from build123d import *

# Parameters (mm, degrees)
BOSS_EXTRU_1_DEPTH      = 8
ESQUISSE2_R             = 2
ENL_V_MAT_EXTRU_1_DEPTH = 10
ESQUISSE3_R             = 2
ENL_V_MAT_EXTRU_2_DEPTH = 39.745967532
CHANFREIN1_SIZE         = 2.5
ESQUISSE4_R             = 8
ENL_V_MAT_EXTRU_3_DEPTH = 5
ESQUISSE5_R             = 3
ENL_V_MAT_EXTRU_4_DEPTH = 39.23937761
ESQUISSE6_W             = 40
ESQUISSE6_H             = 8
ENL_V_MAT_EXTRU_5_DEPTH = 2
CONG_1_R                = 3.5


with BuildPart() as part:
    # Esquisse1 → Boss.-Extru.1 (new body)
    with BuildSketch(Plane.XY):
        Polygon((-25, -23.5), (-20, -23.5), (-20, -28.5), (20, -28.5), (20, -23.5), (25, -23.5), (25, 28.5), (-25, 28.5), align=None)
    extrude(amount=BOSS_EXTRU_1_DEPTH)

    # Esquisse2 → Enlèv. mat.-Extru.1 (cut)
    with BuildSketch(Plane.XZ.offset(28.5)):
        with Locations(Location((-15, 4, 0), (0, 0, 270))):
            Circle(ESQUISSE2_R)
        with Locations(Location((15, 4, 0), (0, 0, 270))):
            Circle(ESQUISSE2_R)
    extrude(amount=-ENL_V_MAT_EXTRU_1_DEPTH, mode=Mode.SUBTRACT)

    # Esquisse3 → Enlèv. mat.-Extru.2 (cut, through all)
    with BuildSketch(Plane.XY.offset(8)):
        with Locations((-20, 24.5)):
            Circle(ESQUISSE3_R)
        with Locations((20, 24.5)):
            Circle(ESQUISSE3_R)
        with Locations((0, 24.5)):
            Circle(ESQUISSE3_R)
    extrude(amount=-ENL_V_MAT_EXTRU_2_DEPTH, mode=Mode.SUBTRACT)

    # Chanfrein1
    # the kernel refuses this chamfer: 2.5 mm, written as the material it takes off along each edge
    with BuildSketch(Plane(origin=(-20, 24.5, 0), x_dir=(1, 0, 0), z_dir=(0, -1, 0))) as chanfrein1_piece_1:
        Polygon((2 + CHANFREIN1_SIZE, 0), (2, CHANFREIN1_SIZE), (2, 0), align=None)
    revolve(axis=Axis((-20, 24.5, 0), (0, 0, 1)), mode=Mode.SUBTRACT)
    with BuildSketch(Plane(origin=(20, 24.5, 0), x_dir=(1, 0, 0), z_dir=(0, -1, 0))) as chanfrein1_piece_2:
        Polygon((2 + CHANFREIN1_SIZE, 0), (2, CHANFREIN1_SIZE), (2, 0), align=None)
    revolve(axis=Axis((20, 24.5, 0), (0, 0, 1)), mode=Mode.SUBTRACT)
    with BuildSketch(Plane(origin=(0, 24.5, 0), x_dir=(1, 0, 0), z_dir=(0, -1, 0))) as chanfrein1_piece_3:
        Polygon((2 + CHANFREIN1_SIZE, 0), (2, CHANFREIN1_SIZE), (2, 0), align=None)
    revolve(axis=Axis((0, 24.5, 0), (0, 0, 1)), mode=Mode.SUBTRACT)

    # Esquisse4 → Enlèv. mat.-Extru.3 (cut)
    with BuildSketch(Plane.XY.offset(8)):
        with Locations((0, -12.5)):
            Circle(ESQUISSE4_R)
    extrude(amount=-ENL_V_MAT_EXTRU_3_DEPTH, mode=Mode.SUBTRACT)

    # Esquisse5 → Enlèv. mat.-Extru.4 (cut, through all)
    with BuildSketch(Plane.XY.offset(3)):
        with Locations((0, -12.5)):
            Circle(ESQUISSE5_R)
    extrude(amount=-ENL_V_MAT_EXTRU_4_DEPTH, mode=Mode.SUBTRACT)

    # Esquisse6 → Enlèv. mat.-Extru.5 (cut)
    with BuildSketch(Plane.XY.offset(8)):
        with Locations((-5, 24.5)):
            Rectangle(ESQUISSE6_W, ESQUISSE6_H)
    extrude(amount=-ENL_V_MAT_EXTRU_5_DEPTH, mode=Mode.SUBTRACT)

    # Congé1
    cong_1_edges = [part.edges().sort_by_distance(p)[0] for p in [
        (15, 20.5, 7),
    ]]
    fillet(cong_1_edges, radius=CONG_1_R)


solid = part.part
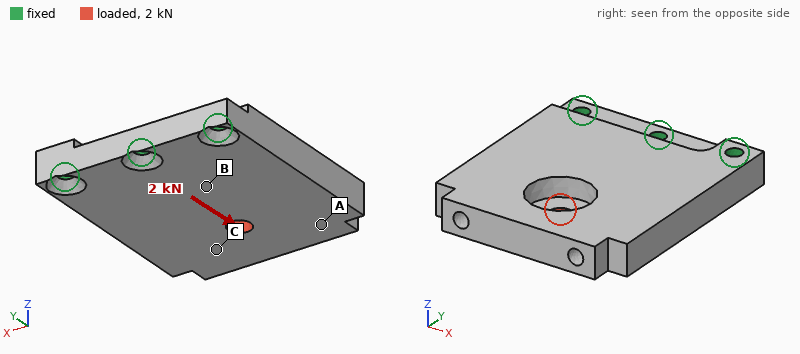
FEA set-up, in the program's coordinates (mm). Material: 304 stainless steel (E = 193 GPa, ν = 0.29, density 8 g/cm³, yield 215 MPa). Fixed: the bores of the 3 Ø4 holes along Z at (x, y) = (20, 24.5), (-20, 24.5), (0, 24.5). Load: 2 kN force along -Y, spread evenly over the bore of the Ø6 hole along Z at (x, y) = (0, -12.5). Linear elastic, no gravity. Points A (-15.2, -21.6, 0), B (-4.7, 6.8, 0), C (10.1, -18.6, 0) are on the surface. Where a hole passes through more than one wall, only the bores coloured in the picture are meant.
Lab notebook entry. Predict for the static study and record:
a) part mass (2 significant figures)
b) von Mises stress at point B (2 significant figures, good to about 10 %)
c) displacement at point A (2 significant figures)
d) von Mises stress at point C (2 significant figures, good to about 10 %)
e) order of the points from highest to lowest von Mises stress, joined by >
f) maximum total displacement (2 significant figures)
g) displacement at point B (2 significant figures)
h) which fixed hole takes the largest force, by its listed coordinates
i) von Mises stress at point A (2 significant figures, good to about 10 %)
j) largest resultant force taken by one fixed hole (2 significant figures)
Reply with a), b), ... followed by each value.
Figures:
a) 160 g
b) 15 MPa
c) 20 µm
d) 11 MPa
e) B > C > A
f) 25 µm
g) 5.7 µm
h) (0, 24.5)
i) 5.5 MPa
j) 770 N
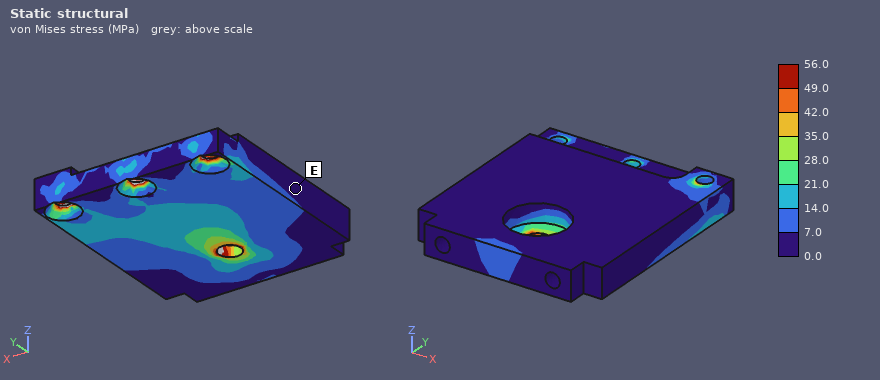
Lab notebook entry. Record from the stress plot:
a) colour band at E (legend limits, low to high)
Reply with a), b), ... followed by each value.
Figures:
a) 0.0 to 7.0 MPa
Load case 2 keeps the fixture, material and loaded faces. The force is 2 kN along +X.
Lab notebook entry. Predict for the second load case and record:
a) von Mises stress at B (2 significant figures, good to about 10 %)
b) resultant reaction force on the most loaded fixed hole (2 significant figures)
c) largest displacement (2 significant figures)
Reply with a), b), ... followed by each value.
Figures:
a) 18 MPa
b) 2.0 kN
c) 14 µm
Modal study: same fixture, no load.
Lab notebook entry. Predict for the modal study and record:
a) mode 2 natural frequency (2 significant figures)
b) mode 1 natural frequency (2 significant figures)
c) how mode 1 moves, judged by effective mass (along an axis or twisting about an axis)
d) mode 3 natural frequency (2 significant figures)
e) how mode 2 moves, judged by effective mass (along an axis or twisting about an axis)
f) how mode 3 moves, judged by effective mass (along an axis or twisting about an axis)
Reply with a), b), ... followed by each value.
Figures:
a) 5100 Hz
b) 1700 Hz
c) along Z
d) 9000 Hz
e) twisting about Y
f) along X
